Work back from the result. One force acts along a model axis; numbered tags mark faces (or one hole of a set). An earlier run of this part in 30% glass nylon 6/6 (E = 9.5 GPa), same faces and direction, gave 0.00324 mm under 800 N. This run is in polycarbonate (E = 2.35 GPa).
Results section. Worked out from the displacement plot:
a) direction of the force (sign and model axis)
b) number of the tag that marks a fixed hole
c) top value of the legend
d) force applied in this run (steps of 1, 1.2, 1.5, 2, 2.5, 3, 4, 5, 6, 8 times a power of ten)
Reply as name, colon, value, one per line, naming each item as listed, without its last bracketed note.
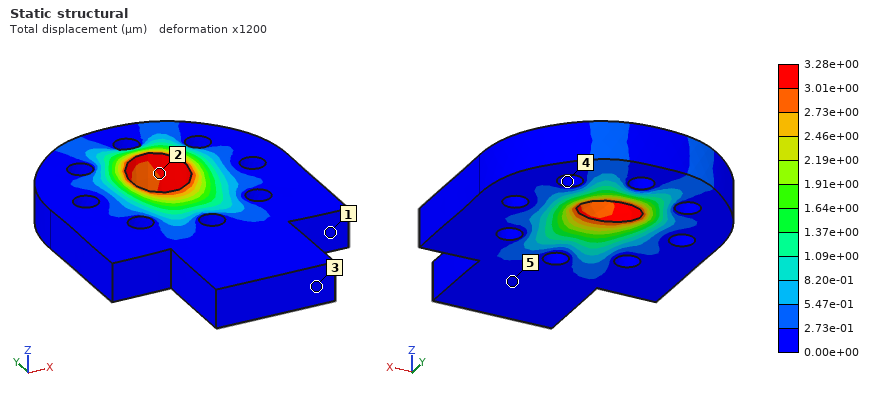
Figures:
direction of the force: +Y
number of the tag that marks a fixed hole: 4
top value of the legend: 3.28e+00 µm
force applied in this run: 200 N
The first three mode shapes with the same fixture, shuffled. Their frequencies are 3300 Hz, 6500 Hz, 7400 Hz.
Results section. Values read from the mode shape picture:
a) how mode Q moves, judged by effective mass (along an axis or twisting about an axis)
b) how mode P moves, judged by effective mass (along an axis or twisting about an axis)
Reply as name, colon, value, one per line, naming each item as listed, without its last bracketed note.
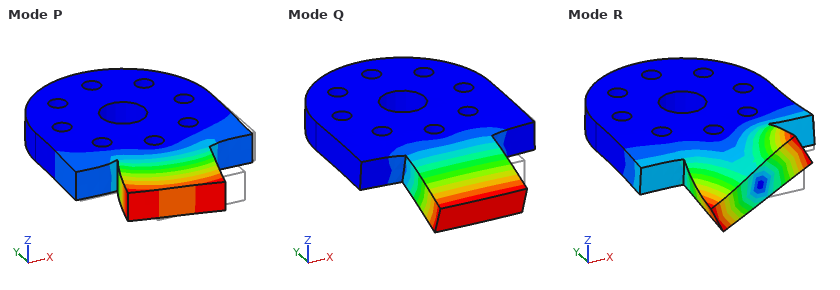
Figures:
how mode Q moves, judged by effective mass: along Z
how mode P moves, judged by effective mass: along X
